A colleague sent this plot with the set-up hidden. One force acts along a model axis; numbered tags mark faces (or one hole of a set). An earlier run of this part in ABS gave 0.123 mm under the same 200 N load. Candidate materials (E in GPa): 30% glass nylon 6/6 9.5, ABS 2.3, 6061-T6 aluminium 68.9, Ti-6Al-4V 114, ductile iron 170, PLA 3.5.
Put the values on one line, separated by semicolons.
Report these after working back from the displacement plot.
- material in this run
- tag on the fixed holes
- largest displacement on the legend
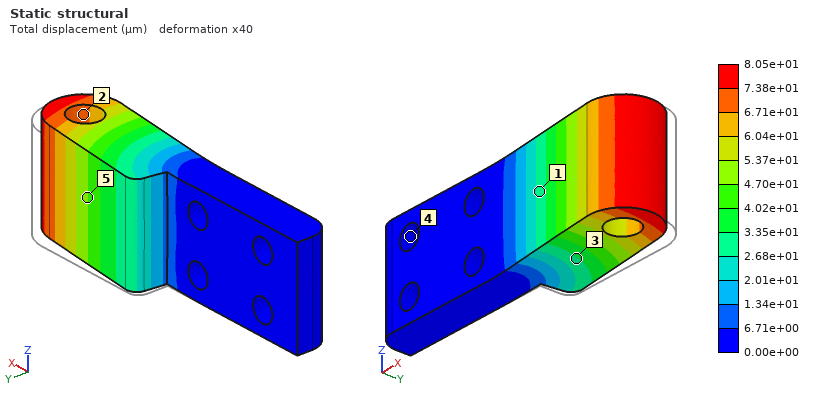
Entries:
PLA; 4; 8.05e+01 µm
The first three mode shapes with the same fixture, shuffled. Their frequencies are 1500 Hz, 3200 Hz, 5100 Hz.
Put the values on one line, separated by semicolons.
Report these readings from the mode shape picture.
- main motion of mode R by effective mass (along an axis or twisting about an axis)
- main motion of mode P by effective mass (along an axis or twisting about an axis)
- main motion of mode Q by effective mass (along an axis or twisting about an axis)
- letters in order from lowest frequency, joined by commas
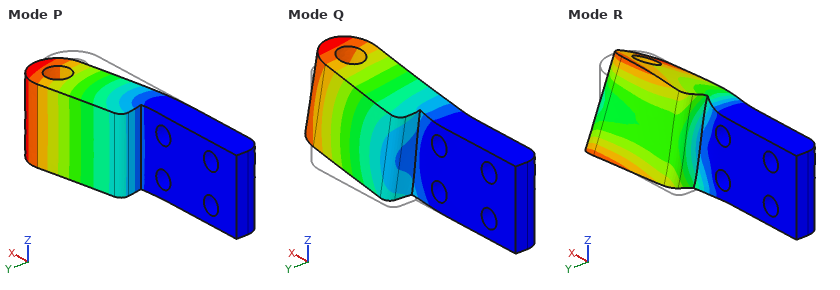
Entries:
twisting about X; along Y; along Z; P, Q, R
